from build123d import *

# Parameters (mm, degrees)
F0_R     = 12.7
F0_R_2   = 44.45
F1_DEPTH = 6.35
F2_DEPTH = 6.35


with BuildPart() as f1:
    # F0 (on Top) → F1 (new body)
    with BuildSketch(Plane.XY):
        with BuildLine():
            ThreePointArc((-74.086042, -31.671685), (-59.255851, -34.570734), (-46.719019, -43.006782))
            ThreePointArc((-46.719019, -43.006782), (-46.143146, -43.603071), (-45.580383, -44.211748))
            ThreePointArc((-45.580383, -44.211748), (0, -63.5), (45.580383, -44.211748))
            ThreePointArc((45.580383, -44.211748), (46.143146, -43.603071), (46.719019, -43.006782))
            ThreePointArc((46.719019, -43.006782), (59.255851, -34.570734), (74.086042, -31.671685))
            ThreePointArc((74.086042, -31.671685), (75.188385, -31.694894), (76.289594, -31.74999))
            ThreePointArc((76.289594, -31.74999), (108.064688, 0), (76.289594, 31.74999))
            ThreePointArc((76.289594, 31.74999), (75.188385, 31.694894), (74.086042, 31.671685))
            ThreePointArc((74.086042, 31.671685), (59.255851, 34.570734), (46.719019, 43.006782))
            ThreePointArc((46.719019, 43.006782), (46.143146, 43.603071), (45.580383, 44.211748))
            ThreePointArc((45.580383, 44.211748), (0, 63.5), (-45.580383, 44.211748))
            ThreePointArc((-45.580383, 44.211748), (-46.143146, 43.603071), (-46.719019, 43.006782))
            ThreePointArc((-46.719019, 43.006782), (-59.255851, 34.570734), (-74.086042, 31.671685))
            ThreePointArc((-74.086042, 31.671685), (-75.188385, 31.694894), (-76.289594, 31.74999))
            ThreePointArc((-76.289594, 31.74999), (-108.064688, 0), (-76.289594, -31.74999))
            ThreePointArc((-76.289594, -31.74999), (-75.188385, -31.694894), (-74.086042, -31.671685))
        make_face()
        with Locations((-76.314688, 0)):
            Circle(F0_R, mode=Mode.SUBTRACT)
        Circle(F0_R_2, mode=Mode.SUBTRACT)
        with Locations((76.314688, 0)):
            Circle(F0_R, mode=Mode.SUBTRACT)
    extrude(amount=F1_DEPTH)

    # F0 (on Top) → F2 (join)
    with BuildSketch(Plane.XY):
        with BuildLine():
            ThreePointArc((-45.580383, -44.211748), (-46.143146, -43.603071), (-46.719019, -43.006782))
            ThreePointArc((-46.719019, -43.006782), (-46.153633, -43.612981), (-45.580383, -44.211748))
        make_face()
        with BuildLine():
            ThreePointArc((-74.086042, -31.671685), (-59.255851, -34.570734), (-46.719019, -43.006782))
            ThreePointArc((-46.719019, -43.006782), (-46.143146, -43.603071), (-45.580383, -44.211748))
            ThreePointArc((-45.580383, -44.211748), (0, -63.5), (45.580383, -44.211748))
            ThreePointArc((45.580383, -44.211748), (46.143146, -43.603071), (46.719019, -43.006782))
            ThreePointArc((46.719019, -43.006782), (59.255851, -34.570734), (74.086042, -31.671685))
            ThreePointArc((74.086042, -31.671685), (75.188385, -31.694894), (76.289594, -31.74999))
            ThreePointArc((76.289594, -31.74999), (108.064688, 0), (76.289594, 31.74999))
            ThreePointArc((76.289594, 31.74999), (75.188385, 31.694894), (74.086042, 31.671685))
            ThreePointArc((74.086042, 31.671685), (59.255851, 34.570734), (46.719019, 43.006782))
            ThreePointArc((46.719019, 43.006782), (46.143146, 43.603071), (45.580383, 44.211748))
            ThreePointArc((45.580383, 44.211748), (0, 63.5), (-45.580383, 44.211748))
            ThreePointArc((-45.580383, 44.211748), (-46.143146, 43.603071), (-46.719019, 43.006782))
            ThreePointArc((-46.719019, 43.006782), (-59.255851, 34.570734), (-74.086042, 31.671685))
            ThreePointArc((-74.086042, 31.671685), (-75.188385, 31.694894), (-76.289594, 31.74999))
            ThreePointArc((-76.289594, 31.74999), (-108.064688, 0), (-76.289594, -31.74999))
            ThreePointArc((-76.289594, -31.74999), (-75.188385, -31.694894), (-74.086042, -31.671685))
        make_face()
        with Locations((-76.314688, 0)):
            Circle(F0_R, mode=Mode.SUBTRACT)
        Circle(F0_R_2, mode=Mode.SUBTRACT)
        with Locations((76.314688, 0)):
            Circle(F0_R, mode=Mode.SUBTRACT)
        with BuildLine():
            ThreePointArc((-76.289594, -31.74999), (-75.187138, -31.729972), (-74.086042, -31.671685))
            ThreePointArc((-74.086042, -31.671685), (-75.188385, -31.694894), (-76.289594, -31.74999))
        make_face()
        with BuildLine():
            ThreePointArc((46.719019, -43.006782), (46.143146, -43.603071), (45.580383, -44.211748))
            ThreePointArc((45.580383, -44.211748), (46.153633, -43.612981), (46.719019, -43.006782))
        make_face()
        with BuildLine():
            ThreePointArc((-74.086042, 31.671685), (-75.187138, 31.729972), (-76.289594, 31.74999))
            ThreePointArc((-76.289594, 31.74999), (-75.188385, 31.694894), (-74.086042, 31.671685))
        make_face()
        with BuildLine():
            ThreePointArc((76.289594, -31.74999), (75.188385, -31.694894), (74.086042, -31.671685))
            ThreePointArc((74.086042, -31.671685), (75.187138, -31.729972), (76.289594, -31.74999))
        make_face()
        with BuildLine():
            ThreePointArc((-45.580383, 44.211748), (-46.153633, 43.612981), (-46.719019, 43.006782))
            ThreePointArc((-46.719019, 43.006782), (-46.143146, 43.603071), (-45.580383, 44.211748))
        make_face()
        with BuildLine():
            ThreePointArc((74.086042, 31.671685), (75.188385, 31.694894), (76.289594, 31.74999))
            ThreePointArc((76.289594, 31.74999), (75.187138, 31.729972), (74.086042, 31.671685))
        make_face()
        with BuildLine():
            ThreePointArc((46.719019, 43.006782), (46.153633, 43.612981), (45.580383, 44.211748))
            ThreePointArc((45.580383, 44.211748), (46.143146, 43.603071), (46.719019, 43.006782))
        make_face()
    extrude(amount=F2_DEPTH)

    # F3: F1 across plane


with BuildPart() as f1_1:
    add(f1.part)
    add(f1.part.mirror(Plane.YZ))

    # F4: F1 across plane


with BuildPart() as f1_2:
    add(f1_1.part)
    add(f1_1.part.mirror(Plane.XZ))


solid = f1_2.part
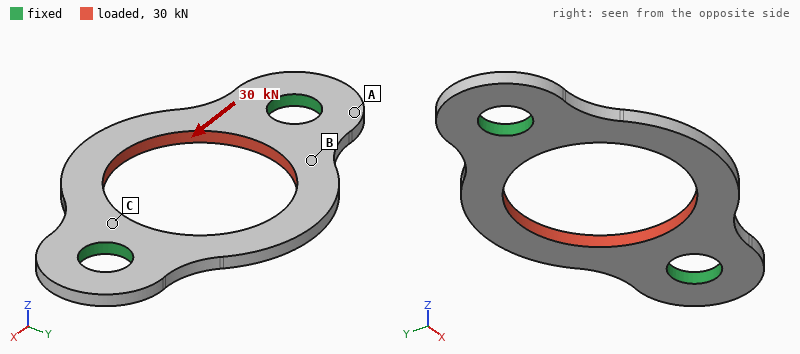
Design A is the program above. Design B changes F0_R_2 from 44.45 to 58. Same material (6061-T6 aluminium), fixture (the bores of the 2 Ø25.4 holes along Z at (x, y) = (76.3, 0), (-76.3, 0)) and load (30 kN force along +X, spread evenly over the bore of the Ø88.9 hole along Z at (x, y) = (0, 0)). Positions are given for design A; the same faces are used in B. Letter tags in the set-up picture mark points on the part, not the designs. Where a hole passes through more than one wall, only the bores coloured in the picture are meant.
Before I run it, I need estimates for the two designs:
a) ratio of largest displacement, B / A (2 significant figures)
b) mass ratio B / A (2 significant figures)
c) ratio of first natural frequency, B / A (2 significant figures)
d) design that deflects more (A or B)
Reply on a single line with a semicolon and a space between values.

13; 0.59; 1.1; B
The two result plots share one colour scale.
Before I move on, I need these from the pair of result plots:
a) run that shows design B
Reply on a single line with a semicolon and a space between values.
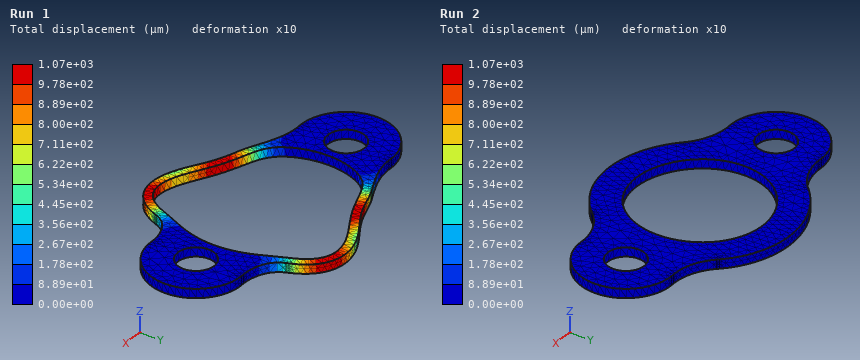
Run 1
